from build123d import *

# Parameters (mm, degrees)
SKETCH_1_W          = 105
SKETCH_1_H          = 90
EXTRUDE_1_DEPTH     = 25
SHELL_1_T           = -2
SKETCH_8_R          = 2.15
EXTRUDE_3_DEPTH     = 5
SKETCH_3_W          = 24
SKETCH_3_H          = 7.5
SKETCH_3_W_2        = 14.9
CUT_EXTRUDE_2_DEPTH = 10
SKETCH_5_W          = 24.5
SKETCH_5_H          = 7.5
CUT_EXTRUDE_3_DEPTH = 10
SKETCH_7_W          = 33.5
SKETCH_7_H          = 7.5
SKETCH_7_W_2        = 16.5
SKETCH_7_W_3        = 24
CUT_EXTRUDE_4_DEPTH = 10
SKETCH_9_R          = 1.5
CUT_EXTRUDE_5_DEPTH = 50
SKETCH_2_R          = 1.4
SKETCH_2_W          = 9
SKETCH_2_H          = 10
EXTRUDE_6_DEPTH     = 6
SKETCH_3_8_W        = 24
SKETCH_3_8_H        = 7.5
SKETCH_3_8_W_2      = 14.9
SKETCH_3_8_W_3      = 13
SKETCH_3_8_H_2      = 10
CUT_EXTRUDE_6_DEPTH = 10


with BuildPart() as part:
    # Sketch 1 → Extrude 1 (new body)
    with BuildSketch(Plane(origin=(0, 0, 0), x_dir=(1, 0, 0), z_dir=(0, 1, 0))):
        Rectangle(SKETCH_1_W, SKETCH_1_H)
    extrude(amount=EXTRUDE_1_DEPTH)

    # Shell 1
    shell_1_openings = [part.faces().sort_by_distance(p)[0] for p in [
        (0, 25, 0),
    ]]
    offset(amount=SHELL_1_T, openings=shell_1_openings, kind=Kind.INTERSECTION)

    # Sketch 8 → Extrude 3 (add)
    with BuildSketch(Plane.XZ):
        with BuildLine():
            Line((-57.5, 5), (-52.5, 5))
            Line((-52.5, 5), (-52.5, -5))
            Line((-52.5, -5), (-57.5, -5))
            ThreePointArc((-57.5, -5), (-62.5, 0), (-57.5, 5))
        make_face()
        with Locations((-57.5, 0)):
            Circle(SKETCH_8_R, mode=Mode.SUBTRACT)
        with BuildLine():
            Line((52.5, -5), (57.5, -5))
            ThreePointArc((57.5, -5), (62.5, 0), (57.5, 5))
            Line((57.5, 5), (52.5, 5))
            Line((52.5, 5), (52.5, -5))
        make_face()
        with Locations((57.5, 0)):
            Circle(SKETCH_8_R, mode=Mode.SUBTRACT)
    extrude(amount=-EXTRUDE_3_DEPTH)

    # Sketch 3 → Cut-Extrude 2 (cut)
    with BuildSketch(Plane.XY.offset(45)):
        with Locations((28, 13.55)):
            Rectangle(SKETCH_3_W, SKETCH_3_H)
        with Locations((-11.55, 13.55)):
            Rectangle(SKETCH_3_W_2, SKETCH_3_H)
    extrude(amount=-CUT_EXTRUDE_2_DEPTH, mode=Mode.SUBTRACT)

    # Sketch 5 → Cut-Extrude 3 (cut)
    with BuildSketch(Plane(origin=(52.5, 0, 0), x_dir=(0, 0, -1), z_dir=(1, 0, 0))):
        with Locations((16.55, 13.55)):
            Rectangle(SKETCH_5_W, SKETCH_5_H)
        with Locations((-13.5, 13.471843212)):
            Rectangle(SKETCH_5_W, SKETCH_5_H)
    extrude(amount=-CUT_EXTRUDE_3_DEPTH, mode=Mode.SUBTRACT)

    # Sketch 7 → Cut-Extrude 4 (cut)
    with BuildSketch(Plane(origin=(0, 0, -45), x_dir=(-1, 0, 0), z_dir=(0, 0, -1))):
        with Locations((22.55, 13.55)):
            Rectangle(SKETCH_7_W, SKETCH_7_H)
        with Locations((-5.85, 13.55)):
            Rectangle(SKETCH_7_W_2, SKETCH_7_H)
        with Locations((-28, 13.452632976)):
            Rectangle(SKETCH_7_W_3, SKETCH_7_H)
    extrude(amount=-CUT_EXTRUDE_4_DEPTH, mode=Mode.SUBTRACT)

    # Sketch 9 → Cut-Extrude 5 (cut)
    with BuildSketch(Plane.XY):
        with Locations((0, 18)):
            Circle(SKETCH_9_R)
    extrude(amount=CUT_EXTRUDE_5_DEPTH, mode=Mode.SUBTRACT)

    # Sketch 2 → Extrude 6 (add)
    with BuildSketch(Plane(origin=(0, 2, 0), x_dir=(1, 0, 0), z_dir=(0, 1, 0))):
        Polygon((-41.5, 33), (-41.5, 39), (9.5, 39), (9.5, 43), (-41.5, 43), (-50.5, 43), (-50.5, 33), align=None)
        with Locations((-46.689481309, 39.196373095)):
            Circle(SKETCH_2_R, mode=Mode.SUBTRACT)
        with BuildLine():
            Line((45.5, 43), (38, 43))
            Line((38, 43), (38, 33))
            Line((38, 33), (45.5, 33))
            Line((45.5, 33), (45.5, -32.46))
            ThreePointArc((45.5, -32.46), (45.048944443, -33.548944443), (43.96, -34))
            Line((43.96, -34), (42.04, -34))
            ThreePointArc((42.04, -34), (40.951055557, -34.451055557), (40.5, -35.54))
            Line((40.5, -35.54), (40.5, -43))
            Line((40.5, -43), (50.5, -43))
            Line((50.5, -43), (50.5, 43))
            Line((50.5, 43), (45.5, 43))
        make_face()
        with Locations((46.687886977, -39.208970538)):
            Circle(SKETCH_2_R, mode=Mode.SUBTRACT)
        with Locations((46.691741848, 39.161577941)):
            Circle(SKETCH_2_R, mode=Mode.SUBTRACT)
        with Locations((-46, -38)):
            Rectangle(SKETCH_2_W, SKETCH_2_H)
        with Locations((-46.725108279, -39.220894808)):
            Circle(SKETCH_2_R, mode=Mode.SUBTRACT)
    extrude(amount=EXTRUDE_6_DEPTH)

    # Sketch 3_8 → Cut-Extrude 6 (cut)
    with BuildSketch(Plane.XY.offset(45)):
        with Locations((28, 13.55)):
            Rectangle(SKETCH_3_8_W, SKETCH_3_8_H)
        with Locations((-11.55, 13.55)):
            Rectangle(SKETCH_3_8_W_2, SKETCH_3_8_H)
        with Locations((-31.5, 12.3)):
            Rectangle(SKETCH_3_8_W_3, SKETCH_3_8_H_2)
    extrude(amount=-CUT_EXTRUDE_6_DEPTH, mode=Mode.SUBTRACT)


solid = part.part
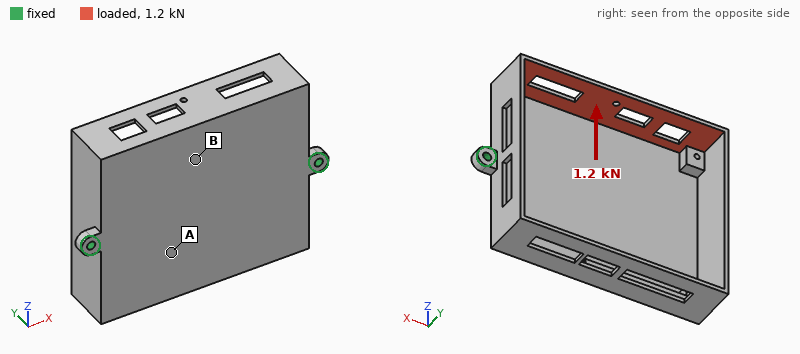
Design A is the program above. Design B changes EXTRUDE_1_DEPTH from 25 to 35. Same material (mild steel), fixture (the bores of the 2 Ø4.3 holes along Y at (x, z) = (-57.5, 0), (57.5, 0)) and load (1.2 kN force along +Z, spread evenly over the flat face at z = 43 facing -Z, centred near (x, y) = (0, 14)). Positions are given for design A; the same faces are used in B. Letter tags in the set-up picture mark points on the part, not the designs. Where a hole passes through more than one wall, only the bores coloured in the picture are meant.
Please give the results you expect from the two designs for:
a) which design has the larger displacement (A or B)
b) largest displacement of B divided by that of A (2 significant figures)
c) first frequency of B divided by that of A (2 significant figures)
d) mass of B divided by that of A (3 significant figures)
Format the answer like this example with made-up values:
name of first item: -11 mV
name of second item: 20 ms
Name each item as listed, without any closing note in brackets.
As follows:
which design has the larger displacement: B
largest displacement of B divided by that of A: 1.6
first frequency of B divided by that of A: 0.86
mass of B divided by that of A: 1.19
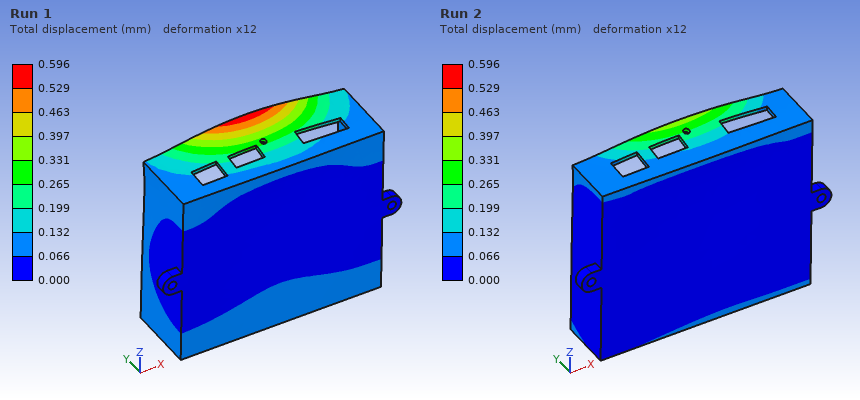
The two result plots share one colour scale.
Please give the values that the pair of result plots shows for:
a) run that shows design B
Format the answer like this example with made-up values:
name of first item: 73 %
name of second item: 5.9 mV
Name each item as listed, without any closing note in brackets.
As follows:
run that shows design B: Run 1
